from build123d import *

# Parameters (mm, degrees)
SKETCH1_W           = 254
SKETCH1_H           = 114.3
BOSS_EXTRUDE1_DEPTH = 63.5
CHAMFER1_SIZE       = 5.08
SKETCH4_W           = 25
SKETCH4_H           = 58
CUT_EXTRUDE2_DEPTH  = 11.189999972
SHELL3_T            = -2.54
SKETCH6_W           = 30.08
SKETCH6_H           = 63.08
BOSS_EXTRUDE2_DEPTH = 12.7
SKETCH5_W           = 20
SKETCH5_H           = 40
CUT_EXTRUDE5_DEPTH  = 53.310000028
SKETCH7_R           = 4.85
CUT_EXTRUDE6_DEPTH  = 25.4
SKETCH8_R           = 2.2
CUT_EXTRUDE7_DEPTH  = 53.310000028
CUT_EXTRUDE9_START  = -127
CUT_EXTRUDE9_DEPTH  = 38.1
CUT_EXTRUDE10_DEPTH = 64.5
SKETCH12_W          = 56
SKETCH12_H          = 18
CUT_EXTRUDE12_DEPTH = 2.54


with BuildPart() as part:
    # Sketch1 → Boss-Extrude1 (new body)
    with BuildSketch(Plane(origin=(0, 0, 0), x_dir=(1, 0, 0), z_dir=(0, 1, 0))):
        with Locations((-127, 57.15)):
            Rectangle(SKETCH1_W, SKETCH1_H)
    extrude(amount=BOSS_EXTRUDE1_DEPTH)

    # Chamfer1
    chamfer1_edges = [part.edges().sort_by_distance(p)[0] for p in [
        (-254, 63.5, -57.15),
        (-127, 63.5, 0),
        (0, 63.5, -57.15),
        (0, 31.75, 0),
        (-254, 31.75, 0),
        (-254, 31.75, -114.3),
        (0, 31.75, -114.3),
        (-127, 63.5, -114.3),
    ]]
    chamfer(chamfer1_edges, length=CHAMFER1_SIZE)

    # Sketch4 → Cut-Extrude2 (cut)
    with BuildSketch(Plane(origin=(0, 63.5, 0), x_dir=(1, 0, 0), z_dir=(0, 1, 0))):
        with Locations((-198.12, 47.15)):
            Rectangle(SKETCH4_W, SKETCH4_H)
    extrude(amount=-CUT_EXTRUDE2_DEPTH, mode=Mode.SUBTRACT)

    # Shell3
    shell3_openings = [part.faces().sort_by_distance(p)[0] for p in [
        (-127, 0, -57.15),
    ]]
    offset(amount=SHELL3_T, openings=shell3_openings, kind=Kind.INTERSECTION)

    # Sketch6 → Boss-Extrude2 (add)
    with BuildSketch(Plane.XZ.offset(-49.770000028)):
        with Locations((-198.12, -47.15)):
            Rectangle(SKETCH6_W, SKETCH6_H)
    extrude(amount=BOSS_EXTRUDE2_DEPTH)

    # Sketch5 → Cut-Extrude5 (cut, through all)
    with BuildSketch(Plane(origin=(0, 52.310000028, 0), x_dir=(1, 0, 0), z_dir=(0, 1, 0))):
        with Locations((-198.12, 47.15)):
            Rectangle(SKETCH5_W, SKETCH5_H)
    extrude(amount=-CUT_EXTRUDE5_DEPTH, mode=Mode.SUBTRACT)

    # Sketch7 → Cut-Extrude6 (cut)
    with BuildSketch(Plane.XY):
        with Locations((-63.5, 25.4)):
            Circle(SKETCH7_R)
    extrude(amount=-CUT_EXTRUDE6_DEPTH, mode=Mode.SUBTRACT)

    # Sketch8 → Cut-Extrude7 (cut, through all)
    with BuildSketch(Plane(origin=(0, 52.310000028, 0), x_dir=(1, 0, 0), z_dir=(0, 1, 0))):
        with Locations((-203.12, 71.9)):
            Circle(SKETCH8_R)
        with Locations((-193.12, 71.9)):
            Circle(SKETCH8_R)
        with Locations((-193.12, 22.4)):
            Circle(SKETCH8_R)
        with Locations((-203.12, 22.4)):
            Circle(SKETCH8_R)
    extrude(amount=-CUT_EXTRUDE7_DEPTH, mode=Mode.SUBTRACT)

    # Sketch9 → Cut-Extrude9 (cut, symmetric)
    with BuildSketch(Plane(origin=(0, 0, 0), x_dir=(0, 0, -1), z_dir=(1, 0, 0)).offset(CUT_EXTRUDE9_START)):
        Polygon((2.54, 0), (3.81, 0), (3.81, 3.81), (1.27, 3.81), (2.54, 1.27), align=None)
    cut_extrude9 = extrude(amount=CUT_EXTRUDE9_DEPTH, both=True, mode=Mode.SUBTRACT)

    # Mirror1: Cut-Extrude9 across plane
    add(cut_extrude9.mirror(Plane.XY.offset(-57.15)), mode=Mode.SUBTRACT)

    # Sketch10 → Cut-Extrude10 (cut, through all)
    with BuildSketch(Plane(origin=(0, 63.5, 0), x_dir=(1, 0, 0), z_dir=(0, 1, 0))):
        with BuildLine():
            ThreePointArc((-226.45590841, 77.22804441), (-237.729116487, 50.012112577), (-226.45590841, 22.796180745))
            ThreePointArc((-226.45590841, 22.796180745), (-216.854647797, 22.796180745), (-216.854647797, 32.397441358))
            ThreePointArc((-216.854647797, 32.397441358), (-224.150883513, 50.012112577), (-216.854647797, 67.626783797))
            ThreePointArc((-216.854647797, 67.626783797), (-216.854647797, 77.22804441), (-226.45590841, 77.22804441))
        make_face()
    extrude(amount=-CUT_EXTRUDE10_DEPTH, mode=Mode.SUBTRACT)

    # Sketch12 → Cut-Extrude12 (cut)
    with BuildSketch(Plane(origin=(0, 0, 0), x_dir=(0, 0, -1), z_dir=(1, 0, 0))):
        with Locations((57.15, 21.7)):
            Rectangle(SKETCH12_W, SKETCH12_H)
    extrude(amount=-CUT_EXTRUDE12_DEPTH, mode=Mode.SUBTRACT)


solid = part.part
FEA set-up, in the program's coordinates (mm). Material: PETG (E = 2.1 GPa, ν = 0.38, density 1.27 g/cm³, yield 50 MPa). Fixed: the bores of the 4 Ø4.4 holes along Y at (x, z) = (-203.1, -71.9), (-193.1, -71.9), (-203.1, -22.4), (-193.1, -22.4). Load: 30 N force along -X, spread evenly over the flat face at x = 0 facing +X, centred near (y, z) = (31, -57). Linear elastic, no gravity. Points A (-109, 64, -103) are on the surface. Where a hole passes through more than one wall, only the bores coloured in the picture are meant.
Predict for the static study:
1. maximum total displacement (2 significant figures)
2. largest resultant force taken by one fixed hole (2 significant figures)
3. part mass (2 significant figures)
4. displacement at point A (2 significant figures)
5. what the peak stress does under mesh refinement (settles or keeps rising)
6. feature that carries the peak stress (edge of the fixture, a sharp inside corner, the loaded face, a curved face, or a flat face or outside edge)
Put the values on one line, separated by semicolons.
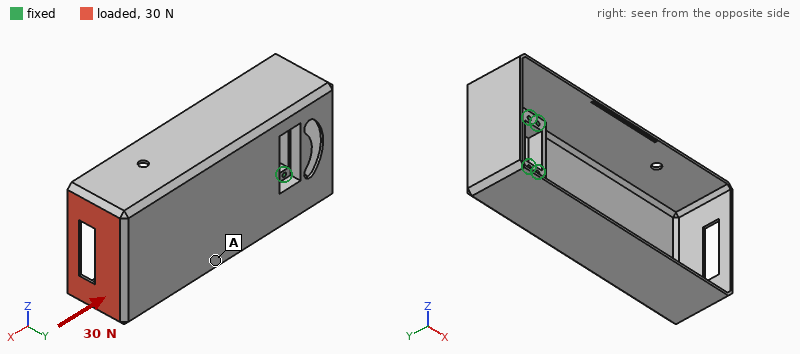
2.7 mm; 23 N; 240 g; 1.0 mm; keeps rising; a sharp inside corner
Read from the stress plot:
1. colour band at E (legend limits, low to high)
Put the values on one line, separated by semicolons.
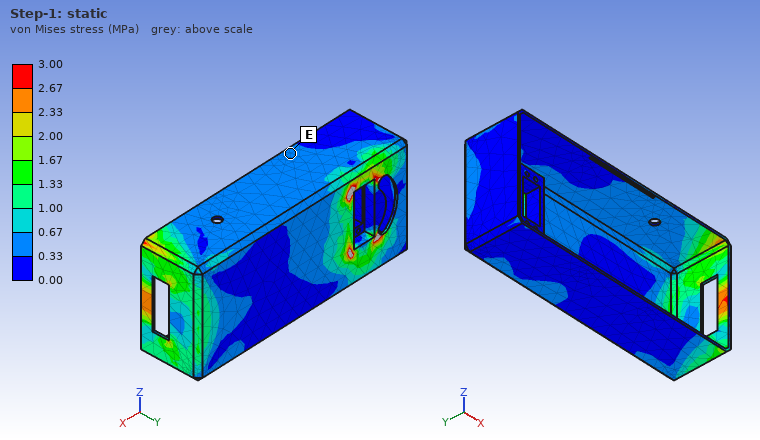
0.33 to 0.67 MPa
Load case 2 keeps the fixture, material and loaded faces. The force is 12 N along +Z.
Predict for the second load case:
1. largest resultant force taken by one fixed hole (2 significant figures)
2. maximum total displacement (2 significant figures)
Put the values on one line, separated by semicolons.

39 N; 3.1 mm
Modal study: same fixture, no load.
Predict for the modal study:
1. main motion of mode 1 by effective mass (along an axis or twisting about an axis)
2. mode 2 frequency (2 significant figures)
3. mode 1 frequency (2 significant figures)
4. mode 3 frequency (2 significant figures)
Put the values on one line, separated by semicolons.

along Y; 44 Hz; 27 Hz; 97 Hz
